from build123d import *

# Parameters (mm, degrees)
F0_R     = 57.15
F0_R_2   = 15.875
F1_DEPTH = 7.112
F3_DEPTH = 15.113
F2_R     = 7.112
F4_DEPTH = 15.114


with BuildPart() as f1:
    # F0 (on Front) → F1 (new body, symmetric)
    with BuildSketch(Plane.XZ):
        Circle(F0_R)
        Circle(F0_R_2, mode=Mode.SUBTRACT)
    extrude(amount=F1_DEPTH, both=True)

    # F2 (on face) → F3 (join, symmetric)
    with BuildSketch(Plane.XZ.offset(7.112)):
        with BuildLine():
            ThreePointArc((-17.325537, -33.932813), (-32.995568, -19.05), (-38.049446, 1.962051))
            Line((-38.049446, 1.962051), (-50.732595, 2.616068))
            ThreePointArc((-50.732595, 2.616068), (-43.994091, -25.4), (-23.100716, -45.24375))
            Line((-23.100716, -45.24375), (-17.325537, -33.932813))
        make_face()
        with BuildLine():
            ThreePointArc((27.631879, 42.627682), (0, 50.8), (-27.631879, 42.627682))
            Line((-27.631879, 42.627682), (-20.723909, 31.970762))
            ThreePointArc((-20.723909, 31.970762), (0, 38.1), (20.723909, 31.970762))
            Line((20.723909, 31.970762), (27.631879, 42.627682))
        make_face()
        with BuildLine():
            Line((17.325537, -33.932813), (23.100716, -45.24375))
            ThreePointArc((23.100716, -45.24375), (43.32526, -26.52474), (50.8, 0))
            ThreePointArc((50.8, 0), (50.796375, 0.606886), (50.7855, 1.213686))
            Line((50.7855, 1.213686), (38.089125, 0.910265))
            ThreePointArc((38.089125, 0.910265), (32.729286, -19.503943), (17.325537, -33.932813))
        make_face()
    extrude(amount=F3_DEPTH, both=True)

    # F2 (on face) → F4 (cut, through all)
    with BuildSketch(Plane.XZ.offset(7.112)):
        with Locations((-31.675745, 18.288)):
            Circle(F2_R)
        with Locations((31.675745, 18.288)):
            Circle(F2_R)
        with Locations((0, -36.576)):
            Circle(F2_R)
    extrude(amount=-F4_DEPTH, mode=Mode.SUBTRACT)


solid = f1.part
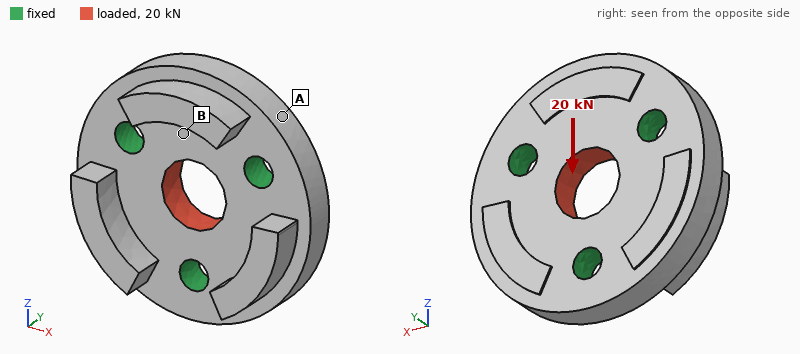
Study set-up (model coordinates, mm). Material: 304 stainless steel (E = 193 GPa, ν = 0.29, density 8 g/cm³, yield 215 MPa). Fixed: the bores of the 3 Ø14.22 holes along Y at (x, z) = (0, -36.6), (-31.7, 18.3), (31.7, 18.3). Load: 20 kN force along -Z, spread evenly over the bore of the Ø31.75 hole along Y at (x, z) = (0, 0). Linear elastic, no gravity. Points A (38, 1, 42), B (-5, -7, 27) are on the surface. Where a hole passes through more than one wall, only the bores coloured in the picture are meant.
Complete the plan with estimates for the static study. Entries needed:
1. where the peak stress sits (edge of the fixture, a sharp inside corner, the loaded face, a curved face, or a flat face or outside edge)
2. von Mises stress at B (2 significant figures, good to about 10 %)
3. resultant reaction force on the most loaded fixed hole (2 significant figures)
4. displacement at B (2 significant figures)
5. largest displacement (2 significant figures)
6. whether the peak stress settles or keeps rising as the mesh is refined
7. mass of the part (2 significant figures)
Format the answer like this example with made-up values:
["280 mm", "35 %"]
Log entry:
["edge of the fixture", "11 MPa", "6.8 kN", "2.2 µm", "3.0 µm", "keeps rising", "1.3 kg"]
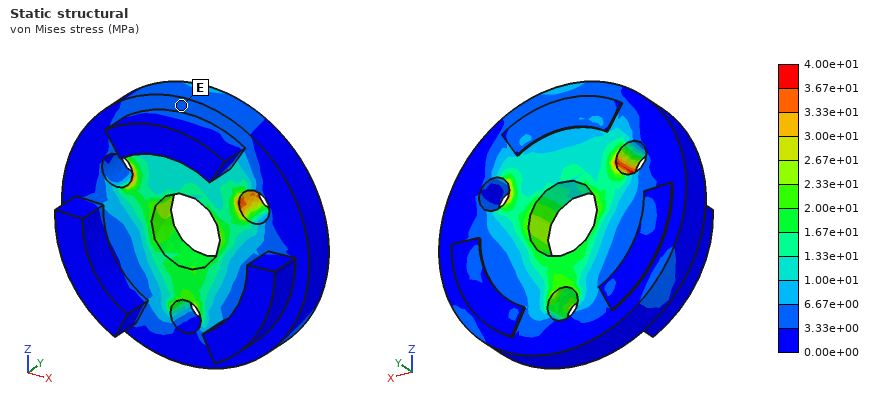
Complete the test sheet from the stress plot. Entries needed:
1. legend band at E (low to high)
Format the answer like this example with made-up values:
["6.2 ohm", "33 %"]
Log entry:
["3.33e+00 to 6.67e+00 MPa"]
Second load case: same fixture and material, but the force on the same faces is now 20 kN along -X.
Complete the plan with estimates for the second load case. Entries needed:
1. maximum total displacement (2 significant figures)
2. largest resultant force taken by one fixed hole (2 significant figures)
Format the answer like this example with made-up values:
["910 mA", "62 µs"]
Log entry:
["2.8 µm", "6.9 kN"]
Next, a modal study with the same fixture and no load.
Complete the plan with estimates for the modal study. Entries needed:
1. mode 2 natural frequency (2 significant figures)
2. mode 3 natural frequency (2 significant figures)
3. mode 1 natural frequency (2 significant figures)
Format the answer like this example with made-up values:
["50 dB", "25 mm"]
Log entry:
["6700 Hz", "6900 Hz", "6700 Hz"]
